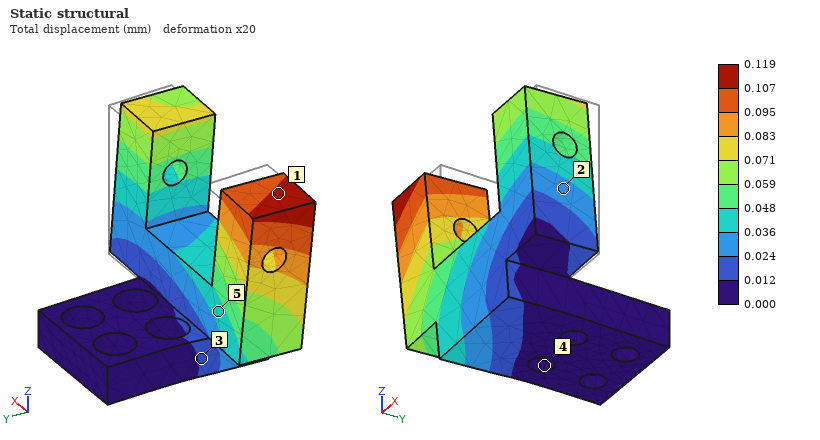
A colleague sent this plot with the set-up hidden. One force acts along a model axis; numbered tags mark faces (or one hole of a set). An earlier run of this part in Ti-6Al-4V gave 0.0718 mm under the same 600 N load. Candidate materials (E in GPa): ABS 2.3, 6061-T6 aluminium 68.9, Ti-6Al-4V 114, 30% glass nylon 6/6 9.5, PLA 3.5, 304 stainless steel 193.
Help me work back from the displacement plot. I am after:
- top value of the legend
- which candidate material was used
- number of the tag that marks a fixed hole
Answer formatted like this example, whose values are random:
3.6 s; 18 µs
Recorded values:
0.119 mm; 6061-T6 aluminium; 4
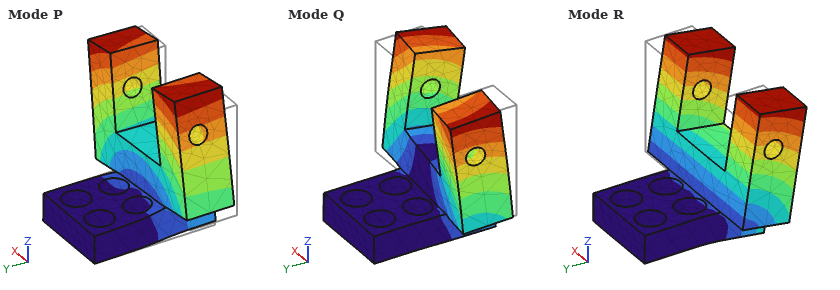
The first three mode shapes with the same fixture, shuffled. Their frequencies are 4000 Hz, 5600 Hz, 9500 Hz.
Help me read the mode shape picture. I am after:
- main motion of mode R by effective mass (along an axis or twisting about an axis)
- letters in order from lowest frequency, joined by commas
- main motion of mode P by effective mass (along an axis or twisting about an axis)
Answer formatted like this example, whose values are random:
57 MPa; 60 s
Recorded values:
along Y; R, P, Q; along X
